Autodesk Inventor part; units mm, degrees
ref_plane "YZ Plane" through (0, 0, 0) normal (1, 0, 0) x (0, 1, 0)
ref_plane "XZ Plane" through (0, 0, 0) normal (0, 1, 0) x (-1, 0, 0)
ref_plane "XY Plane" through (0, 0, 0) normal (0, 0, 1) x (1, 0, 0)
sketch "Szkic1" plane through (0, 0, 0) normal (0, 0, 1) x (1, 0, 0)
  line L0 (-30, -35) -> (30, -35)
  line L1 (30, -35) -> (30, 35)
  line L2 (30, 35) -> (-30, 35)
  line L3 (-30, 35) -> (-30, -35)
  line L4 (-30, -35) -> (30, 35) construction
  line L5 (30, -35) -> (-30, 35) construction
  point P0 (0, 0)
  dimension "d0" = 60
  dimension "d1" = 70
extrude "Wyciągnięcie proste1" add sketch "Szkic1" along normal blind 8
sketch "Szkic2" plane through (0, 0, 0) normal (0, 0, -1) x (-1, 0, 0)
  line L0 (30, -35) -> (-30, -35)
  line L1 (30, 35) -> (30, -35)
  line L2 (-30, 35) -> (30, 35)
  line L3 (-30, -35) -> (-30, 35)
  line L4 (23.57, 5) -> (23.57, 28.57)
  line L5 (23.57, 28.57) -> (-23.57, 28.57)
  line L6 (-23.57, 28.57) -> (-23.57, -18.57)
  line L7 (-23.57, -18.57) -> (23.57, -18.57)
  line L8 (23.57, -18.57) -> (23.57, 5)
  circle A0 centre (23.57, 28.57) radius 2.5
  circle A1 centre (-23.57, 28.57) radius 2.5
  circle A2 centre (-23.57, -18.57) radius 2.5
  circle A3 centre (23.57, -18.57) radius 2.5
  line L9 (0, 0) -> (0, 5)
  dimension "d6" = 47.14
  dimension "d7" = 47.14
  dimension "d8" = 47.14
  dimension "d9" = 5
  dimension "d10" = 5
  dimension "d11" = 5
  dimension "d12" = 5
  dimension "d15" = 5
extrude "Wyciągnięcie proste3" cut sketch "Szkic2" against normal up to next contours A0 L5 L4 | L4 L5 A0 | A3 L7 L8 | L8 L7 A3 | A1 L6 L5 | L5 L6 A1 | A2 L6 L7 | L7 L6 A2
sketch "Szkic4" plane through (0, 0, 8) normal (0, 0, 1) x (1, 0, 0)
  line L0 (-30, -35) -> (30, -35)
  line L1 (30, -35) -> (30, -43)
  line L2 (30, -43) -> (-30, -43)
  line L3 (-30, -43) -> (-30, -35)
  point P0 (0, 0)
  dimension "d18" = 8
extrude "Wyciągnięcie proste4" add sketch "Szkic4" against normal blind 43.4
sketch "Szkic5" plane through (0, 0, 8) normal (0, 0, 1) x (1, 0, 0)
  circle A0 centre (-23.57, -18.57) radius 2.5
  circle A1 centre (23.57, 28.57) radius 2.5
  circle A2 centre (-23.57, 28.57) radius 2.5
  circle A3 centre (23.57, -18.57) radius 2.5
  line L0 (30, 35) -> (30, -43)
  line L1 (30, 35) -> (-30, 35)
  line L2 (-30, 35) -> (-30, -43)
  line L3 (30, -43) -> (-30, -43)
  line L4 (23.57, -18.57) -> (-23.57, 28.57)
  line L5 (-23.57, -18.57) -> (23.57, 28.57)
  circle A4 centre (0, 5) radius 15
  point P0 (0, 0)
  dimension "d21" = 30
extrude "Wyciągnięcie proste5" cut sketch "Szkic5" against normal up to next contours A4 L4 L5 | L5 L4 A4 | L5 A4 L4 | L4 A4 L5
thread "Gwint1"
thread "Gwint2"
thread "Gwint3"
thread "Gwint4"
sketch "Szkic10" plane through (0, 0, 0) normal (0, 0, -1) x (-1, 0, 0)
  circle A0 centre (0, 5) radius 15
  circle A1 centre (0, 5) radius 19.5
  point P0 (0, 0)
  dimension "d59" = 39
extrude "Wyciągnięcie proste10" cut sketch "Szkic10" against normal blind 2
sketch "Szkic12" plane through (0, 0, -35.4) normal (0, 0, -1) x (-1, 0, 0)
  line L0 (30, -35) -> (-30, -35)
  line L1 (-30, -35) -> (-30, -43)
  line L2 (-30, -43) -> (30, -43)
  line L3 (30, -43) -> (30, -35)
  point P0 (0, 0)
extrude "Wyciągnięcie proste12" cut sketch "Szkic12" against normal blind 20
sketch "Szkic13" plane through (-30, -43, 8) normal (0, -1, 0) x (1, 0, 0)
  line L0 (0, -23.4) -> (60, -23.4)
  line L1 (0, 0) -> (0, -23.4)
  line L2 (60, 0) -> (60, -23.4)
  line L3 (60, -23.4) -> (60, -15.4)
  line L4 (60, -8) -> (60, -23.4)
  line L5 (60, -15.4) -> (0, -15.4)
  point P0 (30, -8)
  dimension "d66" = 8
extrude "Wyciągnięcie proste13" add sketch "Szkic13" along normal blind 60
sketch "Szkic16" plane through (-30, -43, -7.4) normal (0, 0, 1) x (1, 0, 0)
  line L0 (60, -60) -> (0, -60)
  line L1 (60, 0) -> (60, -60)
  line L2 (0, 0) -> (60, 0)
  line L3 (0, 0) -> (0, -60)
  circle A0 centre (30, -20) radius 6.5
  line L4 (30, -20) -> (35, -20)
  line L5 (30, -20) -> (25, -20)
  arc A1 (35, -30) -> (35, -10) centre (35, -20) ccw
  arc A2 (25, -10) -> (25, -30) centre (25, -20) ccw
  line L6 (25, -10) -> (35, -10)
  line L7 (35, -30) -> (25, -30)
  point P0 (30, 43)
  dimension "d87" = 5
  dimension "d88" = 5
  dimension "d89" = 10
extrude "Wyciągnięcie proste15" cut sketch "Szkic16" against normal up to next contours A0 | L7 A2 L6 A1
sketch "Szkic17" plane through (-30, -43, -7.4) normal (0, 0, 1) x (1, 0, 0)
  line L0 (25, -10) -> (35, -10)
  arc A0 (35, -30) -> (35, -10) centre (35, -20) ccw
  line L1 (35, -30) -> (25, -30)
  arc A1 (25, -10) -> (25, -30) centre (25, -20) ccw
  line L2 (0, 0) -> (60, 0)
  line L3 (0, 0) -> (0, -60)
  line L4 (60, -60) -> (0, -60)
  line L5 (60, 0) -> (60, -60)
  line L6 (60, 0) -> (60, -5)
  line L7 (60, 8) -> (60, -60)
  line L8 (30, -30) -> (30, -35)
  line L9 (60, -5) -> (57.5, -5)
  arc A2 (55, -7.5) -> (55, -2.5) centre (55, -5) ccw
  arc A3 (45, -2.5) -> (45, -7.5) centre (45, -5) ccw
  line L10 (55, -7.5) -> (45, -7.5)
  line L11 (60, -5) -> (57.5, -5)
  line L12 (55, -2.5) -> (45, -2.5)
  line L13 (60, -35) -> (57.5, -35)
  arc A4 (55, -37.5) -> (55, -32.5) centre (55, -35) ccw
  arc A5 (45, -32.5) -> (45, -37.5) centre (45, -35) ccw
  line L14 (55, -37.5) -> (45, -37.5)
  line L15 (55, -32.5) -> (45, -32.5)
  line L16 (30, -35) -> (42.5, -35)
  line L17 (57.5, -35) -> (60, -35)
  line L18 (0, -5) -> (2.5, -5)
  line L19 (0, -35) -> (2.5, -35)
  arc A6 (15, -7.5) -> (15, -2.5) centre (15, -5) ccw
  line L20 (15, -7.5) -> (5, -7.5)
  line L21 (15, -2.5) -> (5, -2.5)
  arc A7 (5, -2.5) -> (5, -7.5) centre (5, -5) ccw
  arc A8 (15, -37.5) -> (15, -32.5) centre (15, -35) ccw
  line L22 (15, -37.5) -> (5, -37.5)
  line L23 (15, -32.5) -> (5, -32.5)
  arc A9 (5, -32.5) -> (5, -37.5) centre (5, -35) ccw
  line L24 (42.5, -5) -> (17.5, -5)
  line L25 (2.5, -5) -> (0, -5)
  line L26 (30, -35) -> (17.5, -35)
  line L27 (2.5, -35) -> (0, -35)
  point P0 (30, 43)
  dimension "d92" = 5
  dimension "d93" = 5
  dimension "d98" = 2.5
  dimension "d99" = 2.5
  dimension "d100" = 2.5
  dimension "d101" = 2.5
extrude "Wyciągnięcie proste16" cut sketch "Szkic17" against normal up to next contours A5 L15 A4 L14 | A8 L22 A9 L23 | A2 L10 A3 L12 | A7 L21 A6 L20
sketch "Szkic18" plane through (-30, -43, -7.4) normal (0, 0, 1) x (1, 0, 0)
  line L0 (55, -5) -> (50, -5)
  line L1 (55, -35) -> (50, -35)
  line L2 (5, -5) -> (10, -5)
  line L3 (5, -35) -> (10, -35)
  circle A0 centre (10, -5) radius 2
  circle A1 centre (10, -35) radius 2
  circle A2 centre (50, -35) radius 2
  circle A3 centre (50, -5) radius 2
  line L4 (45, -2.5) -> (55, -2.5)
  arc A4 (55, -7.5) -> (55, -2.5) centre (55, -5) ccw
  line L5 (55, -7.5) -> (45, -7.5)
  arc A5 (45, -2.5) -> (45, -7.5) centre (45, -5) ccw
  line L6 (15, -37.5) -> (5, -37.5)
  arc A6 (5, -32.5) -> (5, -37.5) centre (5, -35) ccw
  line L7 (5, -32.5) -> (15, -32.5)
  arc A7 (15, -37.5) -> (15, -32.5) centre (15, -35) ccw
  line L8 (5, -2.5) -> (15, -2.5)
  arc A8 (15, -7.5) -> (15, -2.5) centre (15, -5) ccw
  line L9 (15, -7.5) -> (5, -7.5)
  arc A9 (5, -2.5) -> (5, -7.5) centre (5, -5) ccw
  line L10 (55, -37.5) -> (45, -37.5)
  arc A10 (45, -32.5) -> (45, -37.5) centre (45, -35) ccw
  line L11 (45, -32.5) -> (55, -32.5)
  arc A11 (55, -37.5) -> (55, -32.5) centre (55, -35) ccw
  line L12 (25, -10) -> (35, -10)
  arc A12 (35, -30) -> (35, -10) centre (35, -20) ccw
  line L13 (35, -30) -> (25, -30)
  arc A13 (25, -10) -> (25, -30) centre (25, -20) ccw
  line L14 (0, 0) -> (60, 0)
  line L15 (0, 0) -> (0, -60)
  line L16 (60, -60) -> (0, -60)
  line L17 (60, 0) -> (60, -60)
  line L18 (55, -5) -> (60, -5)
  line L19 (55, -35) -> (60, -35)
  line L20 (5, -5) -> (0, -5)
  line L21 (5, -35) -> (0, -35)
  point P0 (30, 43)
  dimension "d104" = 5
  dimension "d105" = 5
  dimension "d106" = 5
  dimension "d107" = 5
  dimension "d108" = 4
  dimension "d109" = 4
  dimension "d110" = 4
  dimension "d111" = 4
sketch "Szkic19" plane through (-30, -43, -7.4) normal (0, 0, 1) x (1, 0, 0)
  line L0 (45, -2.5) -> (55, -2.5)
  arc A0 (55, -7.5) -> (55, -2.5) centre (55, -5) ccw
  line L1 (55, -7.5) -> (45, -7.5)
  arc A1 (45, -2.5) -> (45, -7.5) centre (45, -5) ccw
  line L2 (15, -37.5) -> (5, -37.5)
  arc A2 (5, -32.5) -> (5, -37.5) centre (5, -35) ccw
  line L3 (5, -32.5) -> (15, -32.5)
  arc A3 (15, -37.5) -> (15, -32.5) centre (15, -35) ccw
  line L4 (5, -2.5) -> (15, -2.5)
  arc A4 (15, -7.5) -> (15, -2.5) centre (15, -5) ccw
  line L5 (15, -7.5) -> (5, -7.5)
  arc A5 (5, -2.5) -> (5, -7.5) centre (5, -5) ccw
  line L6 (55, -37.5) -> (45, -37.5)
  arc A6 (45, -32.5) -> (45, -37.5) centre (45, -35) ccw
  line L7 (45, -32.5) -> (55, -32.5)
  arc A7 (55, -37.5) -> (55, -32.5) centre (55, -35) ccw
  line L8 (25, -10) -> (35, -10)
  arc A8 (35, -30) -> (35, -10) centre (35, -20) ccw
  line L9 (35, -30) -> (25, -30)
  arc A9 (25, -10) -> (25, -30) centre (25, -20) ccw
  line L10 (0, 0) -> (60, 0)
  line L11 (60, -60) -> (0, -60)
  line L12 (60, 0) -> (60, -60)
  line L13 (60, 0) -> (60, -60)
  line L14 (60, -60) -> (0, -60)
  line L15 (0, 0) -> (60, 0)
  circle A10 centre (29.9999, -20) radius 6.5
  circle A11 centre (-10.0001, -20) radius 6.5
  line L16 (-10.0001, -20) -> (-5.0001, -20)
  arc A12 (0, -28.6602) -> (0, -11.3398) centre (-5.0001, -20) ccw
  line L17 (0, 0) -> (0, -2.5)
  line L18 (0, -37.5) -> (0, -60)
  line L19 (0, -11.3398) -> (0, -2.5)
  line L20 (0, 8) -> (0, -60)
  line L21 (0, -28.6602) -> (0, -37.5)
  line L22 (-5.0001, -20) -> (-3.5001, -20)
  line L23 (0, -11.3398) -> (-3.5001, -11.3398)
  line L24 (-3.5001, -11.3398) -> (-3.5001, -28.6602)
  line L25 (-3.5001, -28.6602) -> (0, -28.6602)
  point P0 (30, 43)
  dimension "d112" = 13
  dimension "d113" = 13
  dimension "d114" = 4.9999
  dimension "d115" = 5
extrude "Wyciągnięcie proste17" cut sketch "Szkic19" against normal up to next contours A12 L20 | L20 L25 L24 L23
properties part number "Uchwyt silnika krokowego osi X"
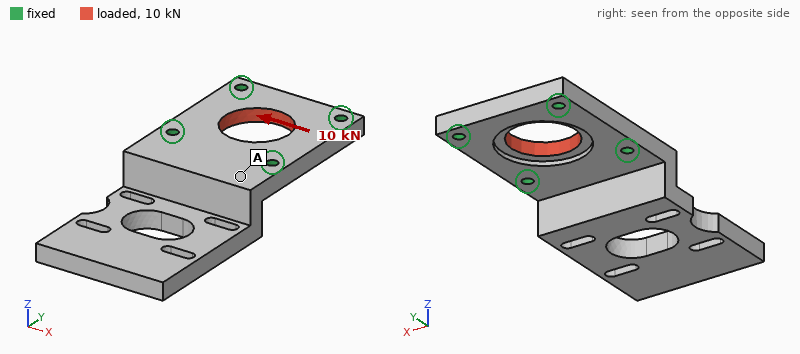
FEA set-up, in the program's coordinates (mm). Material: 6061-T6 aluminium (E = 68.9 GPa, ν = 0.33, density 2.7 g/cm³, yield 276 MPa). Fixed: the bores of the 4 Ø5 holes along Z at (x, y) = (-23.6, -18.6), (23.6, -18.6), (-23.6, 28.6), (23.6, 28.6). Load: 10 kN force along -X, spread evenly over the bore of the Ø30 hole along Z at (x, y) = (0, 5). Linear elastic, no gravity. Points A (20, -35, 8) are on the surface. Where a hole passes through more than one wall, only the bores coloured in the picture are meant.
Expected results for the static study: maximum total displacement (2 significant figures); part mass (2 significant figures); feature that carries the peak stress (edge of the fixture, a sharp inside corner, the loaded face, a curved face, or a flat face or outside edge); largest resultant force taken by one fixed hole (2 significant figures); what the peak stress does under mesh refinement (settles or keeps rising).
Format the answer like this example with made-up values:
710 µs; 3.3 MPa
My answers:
15 µm; 160 g; edge of the fixture; 2.7 kN; keeps rising
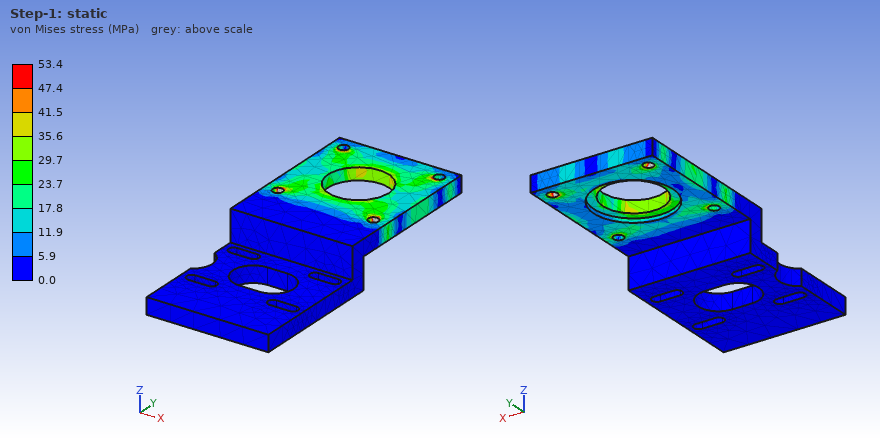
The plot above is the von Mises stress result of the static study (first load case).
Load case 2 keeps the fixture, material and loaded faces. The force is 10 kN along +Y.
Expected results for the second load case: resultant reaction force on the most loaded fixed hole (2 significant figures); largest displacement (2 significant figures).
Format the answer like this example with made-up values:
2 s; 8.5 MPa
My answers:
2.7 kN; 16 µm
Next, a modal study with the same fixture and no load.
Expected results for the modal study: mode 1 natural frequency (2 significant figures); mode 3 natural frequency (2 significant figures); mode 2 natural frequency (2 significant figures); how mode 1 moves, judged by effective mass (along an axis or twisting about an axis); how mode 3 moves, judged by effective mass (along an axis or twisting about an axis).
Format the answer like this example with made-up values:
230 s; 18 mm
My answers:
690 Hz; 3000 Hz; 2300 Hz; along Z; along X
